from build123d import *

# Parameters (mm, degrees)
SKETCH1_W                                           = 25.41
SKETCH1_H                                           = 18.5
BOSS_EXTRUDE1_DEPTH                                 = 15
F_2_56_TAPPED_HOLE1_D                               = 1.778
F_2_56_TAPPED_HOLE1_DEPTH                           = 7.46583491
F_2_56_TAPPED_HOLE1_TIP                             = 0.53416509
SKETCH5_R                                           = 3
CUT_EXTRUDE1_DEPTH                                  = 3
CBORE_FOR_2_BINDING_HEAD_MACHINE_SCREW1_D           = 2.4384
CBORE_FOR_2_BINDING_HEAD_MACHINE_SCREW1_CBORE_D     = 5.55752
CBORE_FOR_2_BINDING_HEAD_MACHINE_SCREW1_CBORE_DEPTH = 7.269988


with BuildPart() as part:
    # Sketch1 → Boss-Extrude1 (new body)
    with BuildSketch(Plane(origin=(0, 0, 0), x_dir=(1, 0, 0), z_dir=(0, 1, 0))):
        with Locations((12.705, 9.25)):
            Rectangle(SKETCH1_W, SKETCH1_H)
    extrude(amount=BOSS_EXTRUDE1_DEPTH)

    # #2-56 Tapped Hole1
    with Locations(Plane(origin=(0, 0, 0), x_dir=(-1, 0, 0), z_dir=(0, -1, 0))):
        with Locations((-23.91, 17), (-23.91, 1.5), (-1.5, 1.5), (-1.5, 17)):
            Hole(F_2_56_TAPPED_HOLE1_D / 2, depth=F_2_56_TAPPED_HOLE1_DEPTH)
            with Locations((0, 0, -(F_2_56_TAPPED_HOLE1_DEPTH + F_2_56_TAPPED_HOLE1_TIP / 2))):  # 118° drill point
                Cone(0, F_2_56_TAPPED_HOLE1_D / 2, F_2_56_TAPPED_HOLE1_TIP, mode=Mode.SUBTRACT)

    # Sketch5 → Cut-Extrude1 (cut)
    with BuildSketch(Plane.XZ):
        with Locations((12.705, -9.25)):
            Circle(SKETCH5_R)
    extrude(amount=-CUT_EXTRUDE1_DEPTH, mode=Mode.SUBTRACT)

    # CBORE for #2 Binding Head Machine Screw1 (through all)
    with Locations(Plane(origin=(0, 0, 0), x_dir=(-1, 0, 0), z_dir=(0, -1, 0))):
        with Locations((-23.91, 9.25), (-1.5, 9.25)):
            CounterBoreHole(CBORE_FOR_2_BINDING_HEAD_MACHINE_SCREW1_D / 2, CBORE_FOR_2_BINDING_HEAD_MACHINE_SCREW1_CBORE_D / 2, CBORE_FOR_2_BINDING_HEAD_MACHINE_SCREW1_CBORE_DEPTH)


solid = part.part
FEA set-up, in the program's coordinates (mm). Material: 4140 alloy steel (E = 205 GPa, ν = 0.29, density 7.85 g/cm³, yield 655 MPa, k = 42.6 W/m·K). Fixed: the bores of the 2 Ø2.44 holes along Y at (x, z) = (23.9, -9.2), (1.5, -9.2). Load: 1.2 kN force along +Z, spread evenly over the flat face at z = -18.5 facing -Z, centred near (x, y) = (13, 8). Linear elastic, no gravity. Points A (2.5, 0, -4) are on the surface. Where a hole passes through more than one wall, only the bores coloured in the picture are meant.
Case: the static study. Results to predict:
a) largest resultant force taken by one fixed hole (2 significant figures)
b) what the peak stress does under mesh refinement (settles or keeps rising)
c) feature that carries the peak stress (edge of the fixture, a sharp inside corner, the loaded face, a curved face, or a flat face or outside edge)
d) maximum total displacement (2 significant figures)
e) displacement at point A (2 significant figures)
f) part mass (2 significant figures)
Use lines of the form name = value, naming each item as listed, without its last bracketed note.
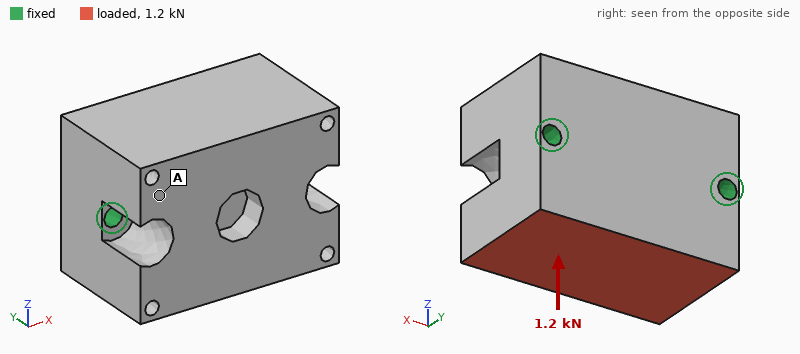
largest resultant force taken by one fixed hole = 600 N
what the peak stress does under mesh refinement = keeps rising
feature that carries the peak stress = edge of the fixture
maximum total displacement = 2.1 µm
displacement at point A = 1.5 µm
part mass = 51 g
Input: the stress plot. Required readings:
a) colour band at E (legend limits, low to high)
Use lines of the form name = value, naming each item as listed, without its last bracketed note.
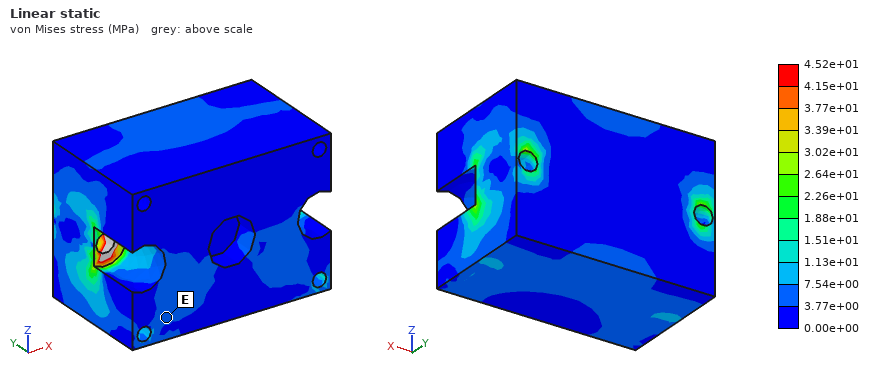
colour band at E = 3.77e+00 to 7.54e+00 MPa
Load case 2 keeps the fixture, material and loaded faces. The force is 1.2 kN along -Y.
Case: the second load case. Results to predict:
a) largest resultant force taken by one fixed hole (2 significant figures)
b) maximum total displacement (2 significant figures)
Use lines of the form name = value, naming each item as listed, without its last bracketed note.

largest resultant force taken by one fixed hole = 610 N
maximum total displacement = 4.7 µm
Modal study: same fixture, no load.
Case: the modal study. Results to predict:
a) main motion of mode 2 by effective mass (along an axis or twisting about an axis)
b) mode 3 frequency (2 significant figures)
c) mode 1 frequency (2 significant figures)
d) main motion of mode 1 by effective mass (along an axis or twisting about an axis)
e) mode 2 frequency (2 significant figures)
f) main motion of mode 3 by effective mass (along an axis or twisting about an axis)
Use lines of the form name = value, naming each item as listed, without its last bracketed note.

main motion of mode 2 by effective mass = along Y
mode 3 frequency = 39 kHz
mode 1 frequency = 19 kHz
main motion of mode 1 by effective mass = along Z
mode 2 frequency = 34 kHz
main motion of mode 3 by effective mass = along X
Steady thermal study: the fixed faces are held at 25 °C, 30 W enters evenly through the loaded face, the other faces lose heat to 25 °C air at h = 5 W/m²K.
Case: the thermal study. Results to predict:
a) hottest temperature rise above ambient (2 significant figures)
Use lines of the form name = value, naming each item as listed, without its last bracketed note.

hottest temperature rise above ambient = 37 K
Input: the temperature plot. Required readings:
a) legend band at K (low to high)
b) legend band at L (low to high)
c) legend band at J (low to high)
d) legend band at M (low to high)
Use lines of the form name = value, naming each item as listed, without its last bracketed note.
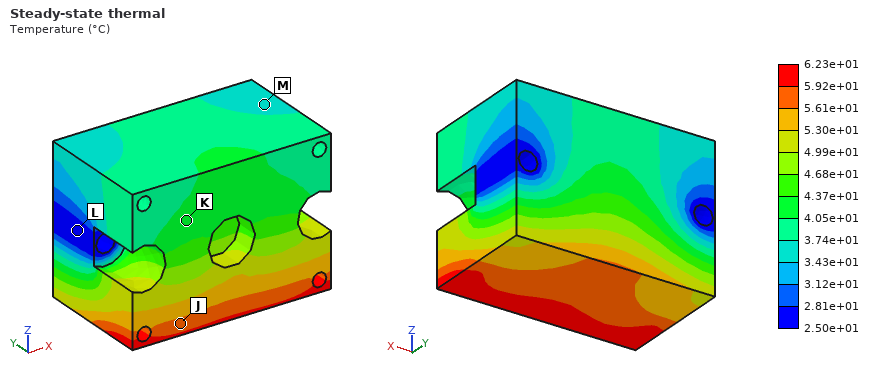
legend band at K = 4.05e+01 to 4.37e+01 °C
legend band at L = 2.50e+01 to 2.81e+01 °C
legend band at J = 5.61e+01 to 5.92e+01 °C
legend band at M = 3.43e+01 to 3.74e+01 °C
